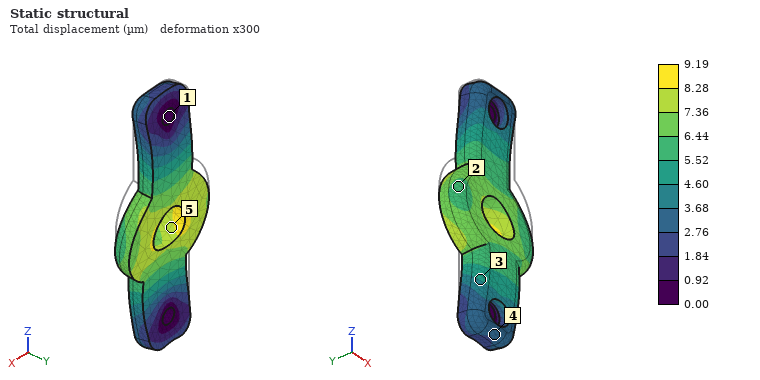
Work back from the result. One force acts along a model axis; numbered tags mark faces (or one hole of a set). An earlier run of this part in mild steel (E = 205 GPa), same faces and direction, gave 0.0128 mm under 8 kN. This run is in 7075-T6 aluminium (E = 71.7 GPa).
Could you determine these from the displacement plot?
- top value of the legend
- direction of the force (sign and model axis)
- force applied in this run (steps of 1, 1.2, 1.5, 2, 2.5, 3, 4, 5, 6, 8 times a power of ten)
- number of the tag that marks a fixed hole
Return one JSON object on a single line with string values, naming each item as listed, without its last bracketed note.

{"top value of the legend": "9.19 µm", "direction of the force": "-Z", "force applied in this run": "2 kN", "number of the tag that marks a fixed hole": "1"}
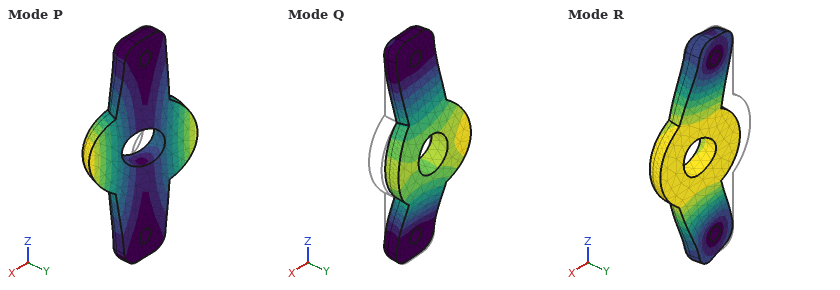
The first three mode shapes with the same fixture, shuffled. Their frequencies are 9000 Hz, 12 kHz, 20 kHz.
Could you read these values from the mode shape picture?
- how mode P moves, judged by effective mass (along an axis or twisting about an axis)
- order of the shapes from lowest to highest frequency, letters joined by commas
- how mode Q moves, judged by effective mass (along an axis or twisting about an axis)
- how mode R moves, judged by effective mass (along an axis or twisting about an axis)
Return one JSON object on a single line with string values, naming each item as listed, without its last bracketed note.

{"how mode P moves, judged by effective mass": "twisting about Z", "order of the shapes from lowest to highest frequency, letters joined by commas": "Q, P, R", "how mode Q moves, judged by effective mass": "along Y", "how mode R moves, judged by effective mass": "along X"}
